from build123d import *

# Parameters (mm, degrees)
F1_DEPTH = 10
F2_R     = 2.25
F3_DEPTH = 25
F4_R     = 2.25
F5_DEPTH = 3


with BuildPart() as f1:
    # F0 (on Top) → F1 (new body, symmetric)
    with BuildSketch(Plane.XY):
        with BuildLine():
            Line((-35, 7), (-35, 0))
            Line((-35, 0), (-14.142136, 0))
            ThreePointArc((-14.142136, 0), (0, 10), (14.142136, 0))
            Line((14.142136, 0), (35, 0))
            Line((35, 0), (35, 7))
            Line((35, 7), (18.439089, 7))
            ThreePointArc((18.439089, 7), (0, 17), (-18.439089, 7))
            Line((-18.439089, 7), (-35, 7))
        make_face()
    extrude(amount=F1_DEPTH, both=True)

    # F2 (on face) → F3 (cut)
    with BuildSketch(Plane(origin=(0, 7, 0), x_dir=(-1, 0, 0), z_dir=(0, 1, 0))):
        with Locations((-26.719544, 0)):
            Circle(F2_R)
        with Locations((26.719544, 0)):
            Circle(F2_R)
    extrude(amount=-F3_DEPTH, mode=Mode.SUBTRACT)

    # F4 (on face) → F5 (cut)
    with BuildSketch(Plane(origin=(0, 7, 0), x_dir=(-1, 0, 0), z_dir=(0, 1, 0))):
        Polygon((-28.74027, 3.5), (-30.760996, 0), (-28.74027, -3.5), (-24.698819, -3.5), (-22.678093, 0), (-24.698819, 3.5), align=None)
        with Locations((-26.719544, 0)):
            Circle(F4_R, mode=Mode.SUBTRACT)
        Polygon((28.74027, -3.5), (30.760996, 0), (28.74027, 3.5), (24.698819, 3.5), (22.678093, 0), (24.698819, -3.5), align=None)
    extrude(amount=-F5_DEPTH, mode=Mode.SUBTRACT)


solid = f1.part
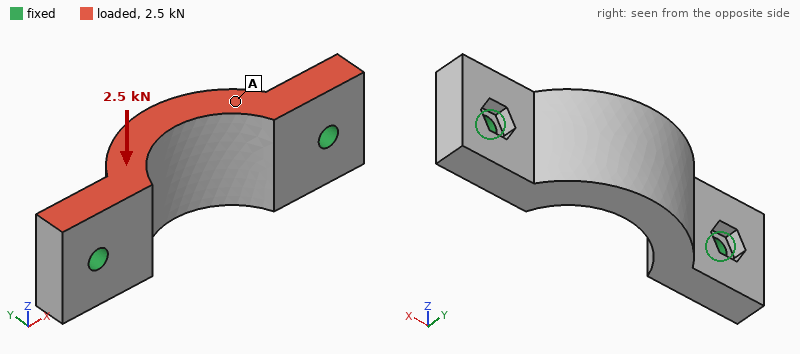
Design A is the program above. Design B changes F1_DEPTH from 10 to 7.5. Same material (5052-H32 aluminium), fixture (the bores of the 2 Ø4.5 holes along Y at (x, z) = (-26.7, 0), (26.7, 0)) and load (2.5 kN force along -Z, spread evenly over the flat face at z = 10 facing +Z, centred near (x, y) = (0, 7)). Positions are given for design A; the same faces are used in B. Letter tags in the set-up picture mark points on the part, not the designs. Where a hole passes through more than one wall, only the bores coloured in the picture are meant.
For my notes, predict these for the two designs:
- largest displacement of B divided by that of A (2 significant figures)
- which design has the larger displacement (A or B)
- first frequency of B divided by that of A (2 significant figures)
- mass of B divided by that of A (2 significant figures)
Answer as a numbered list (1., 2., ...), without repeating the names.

1. 1.1
2. B
3. 1.1
4. 0.74
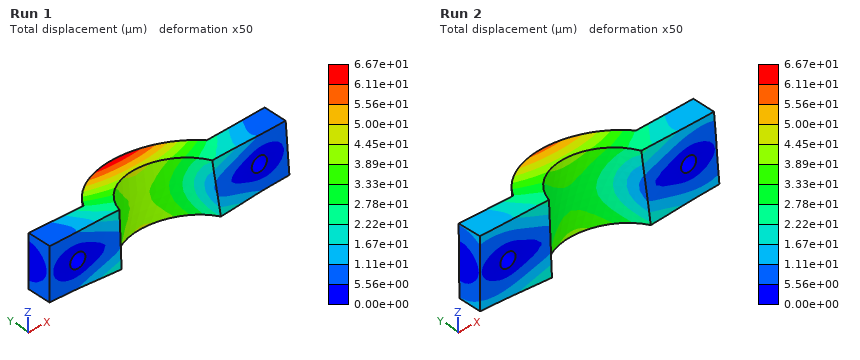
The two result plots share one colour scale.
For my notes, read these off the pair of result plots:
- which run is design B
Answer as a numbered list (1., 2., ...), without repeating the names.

1. Run 1
